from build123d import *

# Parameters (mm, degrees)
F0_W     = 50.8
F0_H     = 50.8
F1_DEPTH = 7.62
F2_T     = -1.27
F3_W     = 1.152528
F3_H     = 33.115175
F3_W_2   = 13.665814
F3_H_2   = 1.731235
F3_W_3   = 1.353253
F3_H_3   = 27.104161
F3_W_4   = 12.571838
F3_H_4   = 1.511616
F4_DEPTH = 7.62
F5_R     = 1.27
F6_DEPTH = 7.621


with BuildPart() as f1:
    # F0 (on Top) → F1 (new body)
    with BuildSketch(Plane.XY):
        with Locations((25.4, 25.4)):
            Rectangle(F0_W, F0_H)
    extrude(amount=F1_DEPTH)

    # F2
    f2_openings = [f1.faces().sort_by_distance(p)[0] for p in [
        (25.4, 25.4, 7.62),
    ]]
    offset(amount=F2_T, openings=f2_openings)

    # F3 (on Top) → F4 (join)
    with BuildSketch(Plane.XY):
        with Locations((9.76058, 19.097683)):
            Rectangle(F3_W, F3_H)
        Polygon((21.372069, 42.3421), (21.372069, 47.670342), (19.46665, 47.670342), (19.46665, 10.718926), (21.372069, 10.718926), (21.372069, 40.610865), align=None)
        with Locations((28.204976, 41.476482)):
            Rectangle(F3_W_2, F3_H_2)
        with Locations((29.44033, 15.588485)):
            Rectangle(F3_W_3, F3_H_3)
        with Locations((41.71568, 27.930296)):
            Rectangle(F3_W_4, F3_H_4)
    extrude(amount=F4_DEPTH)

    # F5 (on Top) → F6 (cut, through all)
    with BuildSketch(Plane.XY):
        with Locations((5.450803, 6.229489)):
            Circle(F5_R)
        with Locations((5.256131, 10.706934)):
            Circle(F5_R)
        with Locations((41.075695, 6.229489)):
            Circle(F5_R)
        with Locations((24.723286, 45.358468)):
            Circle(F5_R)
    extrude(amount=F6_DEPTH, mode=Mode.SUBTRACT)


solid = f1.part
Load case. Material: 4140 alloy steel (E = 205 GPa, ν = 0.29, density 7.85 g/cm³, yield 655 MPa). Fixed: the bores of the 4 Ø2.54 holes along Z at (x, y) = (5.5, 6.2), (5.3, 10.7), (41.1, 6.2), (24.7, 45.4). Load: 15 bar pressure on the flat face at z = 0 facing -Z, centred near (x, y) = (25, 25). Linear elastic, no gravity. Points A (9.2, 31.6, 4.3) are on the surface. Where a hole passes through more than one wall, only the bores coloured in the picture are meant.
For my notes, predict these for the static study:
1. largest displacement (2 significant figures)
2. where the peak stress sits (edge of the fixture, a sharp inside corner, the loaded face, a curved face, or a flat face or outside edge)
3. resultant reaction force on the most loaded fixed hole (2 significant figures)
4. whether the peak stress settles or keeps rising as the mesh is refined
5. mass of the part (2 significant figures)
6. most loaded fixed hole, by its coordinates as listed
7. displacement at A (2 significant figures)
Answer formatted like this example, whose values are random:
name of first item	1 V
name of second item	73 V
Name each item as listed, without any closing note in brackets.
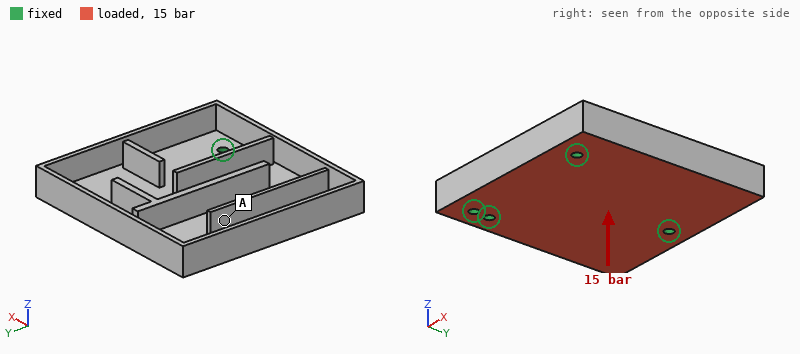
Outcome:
largest displacement	0.22 mm
where the peak stress sits	edge of the fixture
resultant reaction force on the most loaded fixed hole	1.9 kN
whether the peak stress settles or keeps rising as the mesh is refined	keeps rising
mass of the part	47 g
most loaded fixed hole, by its coordinates as listed	(24.7, 45.4)
displacement at A	0.039 mm
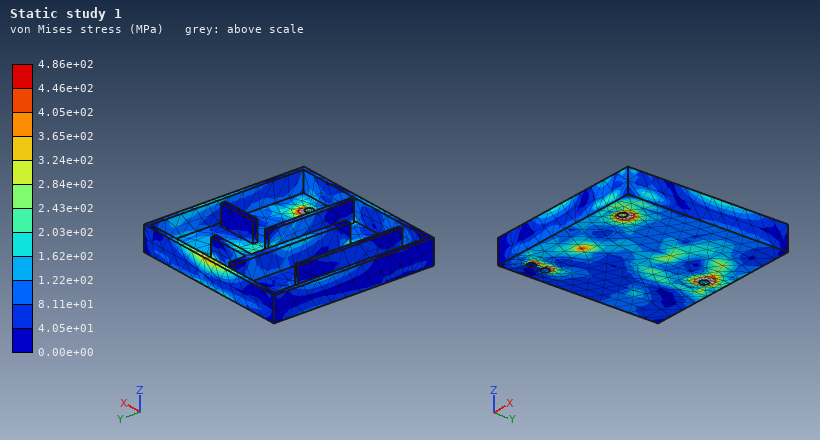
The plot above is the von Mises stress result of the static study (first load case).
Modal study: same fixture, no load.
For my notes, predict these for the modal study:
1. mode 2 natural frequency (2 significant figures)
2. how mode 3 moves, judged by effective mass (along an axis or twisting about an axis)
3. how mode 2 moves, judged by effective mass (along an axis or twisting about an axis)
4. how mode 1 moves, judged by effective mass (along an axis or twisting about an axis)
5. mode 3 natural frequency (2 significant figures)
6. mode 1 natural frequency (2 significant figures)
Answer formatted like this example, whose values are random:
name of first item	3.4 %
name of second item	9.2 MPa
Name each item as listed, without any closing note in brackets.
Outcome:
mode 2 natural frequency	5100 Hz
how mode 3 moves, judged by effective mass	along Z
how mode 2 moves, judged by effective mass	along Z
how mode 1 moves, judged by effective mass	twisting about Y
mode 3 natural frequency	5400 Hz
mode 1 natural frequency	2200 Hz
